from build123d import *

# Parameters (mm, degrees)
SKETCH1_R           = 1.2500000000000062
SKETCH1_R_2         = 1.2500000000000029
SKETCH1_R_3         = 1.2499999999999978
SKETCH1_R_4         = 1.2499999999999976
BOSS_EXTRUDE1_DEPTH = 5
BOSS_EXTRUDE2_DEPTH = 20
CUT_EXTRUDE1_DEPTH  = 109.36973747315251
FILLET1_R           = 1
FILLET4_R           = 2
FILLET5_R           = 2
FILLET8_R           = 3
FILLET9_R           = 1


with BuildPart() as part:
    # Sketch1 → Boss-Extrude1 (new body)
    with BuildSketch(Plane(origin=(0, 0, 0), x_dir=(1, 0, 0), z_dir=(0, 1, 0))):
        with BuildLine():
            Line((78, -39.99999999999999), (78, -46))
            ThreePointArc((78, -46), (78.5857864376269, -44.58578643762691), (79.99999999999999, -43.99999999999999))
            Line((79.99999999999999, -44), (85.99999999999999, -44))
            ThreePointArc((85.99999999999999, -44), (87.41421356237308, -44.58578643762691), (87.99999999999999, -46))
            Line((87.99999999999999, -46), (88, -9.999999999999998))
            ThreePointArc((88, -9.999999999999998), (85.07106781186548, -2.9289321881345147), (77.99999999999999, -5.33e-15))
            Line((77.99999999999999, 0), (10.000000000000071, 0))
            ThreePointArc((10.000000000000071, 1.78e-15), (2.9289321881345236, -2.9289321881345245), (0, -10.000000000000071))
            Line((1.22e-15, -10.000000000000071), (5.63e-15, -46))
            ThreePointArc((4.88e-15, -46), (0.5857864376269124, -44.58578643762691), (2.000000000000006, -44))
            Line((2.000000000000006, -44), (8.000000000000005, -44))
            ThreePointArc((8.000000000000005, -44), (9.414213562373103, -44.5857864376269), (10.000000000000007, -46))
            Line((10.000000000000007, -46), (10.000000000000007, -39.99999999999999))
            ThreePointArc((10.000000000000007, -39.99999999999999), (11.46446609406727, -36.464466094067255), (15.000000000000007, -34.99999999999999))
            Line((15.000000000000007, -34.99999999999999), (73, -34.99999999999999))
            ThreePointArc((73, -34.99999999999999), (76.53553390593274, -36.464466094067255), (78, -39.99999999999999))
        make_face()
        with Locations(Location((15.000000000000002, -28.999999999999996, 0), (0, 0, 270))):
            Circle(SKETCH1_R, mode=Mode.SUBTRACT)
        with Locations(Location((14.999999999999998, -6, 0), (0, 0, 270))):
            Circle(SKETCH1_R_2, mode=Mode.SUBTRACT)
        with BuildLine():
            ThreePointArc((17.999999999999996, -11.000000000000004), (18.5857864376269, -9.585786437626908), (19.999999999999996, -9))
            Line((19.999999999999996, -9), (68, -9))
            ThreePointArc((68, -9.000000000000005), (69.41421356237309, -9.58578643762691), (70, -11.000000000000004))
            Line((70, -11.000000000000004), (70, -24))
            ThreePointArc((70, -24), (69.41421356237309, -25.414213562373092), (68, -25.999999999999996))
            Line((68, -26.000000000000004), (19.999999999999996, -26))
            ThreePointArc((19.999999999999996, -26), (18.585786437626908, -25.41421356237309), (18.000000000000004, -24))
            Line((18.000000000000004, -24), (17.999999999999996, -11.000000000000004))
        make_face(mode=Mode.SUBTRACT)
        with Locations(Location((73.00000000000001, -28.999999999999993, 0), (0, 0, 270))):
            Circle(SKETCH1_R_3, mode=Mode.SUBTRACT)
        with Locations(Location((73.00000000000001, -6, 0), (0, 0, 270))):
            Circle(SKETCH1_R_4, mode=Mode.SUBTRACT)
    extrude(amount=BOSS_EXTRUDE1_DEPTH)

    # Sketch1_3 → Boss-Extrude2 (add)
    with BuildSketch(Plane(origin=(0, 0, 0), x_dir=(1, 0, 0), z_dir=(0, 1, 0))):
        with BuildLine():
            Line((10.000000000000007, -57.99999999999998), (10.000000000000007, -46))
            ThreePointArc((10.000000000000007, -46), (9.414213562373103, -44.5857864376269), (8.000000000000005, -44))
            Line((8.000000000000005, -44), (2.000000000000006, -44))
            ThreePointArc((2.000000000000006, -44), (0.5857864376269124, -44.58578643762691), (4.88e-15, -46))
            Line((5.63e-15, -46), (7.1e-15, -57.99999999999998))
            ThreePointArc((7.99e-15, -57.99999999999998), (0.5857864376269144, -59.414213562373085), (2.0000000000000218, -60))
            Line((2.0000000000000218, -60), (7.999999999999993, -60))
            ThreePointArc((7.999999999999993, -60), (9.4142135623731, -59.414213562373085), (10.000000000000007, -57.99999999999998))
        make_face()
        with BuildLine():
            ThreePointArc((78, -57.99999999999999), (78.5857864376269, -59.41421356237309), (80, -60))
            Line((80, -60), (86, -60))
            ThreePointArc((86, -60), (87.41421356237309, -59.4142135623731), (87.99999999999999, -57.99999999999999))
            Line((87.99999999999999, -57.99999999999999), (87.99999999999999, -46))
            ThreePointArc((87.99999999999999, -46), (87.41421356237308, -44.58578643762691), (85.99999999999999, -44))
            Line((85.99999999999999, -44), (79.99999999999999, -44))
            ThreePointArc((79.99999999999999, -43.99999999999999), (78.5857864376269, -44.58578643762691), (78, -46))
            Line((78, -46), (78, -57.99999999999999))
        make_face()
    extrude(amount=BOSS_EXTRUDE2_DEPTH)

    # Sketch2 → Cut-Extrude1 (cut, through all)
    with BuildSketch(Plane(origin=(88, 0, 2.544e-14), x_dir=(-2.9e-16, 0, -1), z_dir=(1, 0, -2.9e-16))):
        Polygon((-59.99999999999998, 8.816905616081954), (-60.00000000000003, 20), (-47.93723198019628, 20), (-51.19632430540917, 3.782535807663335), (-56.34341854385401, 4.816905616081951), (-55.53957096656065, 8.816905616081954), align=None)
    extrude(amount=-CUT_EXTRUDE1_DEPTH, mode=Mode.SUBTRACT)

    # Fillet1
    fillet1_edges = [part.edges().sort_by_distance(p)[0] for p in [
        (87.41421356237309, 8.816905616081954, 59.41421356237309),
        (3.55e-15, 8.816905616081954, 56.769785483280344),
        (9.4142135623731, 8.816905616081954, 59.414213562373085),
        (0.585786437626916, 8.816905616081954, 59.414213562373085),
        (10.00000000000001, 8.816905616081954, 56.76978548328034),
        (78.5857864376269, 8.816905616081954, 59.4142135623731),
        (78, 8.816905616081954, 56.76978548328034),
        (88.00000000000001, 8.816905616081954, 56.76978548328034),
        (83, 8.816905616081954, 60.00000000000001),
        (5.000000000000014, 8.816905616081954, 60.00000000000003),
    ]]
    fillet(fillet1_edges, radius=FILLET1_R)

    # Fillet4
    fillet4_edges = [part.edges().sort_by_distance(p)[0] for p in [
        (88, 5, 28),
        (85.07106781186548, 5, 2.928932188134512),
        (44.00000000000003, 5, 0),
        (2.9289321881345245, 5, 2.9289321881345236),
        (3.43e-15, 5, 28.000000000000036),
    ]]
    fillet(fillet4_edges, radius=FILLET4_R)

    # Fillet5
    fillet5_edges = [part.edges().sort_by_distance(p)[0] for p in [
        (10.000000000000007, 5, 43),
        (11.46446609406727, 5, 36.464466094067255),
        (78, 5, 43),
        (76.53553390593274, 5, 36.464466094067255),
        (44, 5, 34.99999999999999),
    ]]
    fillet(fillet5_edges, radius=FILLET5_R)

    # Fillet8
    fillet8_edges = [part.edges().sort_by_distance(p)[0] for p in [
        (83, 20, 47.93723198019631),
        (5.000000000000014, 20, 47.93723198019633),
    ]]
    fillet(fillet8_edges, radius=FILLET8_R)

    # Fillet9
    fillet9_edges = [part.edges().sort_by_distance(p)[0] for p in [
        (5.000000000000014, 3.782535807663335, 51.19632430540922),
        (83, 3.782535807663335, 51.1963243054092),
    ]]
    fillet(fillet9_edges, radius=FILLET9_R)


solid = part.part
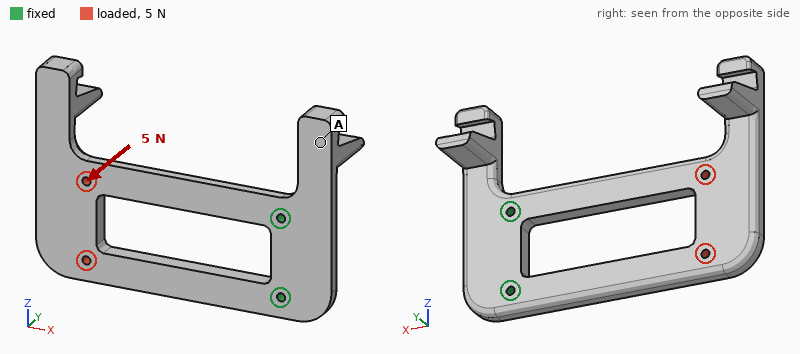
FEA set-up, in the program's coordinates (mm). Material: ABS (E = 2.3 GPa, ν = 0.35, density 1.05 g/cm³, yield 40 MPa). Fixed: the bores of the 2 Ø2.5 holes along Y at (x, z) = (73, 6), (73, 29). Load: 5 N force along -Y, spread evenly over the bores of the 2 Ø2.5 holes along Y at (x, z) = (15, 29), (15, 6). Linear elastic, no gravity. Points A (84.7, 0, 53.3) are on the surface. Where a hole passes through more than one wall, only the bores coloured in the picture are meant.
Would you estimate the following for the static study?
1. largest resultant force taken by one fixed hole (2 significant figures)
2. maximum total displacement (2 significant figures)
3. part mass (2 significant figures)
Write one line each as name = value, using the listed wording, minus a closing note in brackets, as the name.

largest resultant force taken by one fixed hole = 2.6 N
maximum total displacement = 1.1 mm
part mass = 16 g
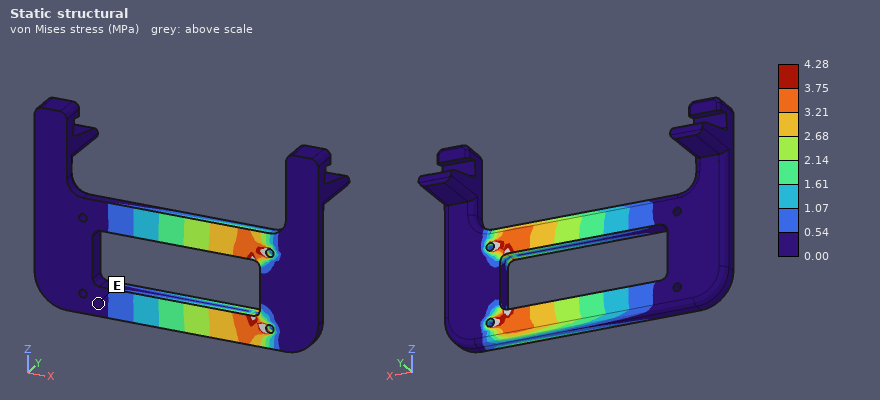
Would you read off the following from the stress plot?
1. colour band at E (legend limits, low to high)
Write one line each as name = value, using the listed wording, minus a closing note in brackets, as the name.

colour band at E = 0.00 to 0.54 MPa
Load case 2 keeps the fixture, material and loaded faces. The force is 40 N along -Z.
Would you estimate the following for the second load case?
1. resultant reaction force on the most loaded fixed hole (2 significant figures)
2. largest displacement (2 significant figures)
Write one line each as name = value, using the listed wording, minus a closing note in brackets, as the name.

resultant reaction force on the most loaded fixed hole = 87 N
largest displacement = 0.69 mm
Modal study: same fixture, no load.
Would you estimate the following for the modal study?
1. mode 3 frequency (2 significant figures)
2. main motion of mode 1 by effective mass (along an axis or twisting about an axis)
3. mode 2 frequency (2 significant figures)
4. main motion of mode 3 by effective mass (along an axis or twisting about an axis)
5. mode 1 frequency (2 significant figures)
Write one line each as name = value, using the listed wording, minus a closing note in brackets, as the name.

mode 3 frequency = 460 Hz
main motion of mode 1 by effective mass = along Y
mode 2 frequency = 350 Hz
main motion of mode 3 by effective mass = along Z
mode 1 frequency = 130 Hz
